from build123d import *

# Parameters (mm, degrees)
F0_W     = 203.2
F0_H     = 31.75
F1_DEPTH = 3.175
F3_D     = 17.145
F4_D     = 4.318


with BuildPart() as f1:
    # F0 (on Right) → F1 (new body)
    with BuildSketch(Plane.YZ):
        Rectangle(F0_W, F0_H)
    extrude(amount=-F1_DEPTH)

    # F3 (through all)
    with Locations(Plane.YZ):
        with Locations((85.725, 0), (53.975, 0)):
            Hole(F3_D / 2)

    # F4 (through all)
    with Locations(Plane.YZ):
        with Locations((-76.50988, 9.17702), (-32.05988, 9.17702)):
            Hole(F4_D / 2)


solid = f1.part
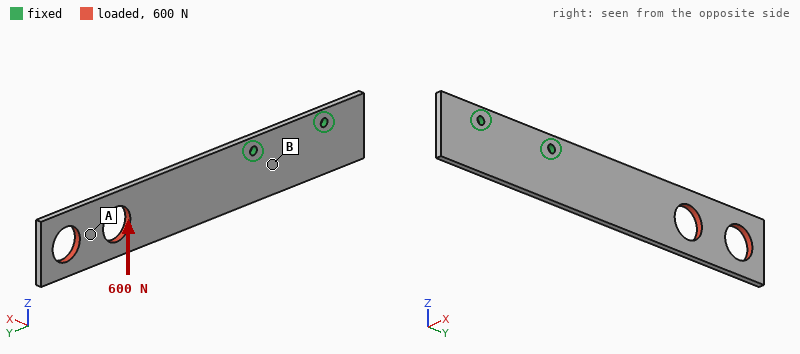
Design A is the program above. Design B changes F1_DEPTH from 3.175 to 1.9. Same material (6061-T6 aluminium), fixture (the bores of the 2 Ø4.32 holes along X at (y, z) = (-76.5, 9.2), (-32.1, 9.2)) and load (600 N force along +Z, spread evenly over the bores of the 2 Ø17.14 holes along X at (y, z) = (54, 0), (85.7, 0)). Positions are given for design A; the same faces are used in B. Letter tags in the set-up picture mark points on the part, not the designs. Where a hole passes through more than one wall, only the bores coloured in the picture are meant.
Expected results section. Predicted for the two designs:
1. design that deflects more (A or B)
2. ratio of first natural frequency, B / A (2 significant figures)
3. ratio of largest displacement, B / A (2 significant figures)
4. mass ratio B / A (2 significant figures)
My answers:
B
0.60
1.7
0.60
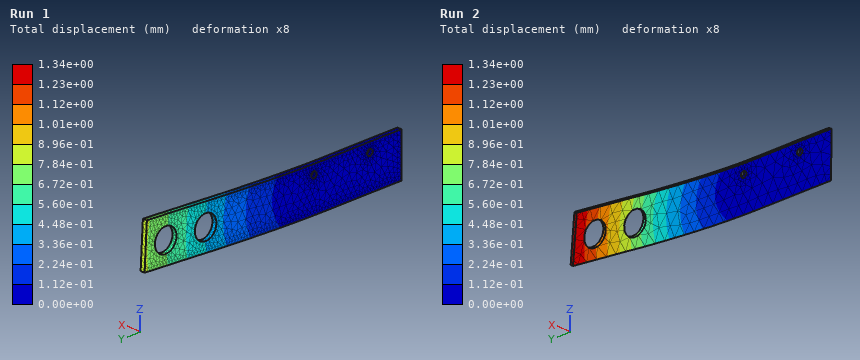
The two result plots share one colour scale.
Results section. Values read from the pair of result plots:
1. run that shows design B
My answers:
Run 2
